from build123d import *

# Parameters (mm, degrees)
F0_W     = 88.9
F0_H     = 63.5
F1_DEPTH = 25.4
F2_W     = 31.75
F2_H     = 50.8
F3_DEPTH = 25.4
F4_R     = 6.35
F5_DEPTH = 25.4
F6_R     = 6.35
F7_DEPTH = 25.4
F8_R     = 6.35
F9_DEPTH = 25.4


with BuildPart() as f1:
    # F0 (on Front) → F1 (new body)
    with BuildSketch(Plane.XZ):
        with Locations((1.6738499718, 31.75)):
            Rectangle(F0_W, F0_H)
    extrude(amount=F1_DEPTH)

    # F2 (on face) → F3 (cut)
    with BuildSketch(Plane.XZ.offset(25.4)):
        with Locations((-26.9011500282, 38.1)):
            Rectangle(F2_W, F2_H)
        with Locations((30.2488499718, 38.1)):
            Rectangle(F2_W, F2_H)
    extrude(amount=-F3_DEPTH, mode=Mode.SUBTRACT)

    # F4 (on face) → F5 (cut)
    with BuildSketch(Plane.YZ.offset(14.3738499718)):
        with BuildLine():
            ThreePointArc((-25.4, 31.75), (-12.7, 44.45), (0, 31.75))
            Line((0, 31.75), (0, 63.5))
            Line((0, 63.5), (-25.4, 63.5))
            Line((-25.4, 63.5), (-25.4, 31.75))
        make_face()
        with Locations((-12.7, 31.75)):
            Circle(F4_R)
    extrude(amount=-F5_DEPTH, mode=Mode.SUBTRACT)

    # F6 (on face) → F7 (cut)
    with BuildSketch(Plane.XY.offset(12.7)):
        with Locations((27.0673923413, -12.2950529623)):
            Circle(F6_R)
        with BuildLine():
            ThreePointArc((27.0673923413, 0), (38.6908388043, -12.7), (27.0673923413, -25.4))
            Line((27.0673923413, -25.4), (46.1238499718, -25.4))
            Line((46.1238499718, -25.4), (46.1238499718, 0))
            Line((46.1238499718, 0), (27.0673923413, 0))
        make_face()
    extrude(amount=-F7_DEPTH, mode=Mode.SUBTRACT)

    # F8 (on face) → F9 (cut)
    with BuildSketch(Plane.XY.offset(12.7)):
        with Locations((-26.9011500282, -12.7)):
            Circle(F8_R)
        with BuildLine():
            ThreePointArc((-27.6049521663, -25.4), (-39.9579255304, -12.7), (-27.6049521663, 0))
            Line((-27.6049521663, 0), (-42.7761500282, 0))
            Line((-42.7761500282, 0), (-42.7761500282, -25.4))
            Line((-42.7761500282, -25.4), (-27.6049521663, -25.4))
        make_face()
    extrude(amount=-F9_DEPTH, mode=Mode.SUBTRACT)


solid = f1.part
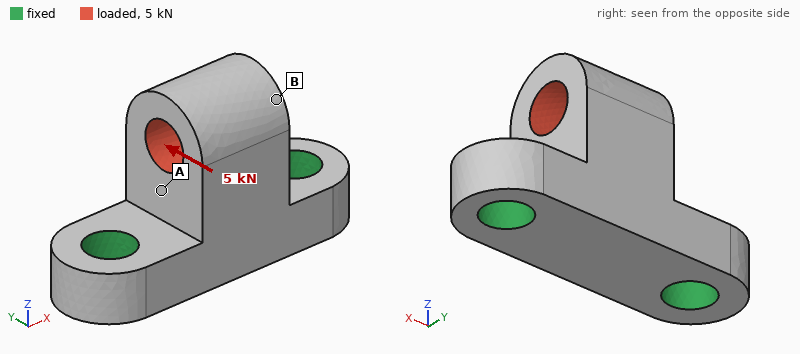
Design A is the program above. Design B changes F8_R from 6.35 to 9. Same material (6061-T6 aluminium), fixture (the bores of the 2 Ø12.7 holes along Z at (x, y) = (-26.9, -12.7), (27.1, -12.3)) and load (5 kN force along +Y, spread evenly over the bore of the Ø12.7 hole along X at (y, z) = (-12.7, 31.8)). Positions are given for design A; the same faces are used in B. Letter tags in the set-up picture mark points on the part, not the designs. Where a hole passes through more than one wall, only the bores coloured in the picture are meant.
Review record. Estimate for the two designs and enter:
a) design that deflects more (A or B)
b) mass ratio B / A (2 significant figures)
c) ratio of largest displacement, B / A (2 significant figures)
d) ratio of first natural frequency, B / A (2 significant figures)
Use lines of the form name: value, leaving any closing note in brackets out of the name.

design that deflects more: A
mass ratio B / A: 0.95
ratio of largest displacement, B / A: 0.90
ratio of first natural frequency, B / A: 1.1
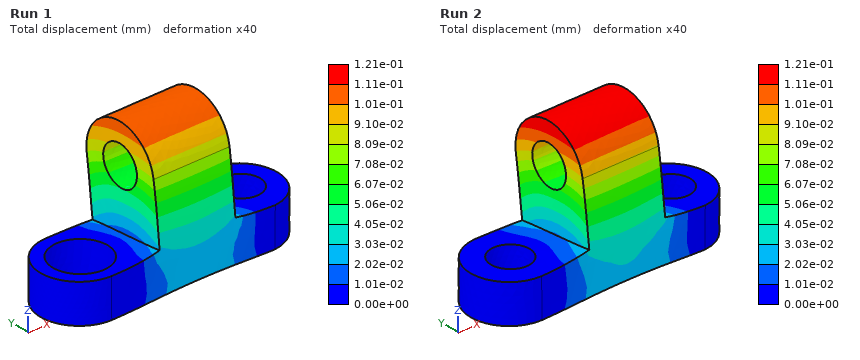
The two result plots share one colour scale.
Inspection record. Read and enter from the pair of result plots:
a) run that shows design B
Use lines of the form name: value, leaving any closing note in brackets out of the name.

run that shows design B: Run 1
